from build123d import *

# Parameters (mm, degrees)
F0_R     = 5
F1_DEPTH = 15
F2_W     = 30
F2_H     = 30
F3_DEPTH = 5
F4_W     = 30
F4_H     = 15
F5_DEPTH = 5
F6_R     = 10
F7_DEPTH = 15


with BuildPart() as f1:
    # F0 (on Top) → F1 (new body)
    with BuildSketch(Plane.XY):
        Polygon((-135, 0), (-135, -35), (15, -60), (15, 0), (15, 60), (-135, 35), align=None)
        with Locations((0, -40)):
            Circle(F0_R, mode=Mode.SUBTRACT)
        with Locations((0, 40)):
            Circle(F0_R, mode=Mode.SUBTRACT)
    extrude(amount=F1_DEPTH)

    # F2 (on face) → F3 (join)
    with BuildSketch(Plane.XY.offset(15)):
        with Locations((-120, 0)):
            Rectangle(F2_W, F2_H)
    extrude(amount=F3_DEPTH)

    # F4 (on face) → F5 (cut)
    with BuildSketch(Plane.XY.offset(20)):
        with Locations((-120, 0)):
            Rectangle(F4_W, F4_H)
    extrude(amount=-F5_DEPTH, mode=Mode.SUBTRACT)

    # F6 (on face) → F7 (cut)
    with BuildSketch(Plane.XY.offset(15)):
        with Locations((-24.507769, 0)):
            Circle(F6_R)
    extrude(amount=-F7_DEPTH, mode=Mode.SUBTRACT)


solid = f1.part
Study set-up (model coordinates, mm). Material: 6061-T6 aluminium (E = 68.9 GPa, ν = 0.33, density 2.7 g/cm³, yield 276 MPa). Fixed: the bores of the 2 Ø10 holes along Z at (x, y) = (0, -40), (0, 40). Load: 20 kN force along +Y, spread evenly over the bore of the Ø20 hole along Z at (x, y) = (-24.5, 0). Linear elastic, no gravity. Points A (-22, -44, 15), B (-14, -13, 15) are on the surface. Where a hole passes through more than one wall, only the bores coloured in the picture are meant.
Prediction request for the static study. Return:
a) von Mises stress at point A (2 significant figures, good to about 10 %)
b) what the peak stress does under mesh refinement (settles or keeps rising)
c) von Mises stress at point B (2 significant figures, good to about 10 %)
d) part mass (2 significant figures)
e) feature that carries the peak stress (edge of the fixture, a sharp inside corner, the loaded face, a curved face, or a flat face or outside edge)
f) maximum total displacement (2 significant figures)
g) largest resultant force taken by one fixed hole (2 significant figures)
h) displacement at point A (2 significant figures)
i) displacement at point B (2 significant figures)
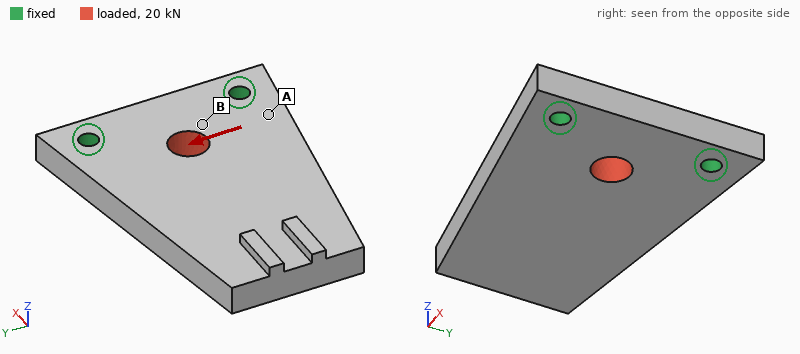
10 MPa
keeps rising
23 MPa
560 g
edge of the fixture
25 µm
11 kN
13 µm
11 µm
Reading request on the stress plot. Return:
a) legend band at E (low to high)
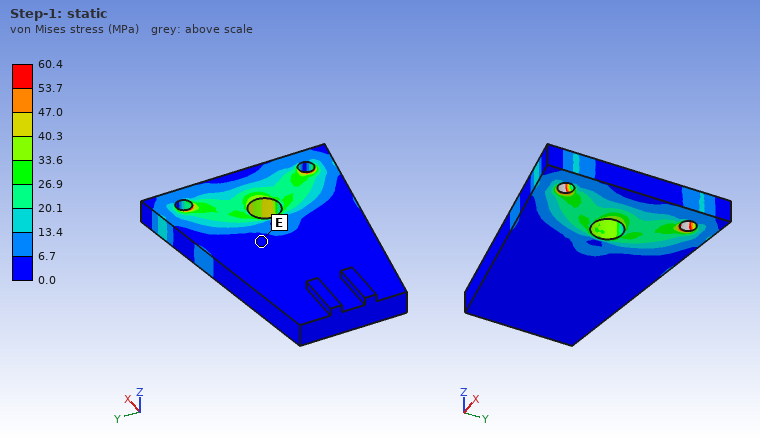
0.0 to 6.7 MPa
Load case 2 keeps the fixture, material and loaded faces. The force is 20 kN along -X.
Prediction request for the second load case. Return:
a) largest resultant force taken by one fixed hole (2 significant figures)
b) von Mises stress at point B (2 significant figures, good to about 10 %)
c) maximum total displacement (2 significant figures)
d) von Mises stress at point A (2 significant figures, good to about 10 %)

10 kN
17 MPa
21 µm
14 MPa
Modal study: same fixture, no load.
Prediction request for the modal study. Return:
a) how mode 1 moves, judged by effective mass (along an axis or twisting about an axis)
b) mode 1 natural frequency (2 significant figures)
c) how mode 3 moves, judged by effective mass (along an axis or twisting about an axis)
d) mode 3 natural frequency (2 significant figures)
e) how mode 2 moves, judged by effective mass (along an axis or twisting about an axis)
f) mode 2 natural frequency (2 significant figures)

along Z
680 Hz
along Y
3700 Hz
twisting about X
2600 Hz
